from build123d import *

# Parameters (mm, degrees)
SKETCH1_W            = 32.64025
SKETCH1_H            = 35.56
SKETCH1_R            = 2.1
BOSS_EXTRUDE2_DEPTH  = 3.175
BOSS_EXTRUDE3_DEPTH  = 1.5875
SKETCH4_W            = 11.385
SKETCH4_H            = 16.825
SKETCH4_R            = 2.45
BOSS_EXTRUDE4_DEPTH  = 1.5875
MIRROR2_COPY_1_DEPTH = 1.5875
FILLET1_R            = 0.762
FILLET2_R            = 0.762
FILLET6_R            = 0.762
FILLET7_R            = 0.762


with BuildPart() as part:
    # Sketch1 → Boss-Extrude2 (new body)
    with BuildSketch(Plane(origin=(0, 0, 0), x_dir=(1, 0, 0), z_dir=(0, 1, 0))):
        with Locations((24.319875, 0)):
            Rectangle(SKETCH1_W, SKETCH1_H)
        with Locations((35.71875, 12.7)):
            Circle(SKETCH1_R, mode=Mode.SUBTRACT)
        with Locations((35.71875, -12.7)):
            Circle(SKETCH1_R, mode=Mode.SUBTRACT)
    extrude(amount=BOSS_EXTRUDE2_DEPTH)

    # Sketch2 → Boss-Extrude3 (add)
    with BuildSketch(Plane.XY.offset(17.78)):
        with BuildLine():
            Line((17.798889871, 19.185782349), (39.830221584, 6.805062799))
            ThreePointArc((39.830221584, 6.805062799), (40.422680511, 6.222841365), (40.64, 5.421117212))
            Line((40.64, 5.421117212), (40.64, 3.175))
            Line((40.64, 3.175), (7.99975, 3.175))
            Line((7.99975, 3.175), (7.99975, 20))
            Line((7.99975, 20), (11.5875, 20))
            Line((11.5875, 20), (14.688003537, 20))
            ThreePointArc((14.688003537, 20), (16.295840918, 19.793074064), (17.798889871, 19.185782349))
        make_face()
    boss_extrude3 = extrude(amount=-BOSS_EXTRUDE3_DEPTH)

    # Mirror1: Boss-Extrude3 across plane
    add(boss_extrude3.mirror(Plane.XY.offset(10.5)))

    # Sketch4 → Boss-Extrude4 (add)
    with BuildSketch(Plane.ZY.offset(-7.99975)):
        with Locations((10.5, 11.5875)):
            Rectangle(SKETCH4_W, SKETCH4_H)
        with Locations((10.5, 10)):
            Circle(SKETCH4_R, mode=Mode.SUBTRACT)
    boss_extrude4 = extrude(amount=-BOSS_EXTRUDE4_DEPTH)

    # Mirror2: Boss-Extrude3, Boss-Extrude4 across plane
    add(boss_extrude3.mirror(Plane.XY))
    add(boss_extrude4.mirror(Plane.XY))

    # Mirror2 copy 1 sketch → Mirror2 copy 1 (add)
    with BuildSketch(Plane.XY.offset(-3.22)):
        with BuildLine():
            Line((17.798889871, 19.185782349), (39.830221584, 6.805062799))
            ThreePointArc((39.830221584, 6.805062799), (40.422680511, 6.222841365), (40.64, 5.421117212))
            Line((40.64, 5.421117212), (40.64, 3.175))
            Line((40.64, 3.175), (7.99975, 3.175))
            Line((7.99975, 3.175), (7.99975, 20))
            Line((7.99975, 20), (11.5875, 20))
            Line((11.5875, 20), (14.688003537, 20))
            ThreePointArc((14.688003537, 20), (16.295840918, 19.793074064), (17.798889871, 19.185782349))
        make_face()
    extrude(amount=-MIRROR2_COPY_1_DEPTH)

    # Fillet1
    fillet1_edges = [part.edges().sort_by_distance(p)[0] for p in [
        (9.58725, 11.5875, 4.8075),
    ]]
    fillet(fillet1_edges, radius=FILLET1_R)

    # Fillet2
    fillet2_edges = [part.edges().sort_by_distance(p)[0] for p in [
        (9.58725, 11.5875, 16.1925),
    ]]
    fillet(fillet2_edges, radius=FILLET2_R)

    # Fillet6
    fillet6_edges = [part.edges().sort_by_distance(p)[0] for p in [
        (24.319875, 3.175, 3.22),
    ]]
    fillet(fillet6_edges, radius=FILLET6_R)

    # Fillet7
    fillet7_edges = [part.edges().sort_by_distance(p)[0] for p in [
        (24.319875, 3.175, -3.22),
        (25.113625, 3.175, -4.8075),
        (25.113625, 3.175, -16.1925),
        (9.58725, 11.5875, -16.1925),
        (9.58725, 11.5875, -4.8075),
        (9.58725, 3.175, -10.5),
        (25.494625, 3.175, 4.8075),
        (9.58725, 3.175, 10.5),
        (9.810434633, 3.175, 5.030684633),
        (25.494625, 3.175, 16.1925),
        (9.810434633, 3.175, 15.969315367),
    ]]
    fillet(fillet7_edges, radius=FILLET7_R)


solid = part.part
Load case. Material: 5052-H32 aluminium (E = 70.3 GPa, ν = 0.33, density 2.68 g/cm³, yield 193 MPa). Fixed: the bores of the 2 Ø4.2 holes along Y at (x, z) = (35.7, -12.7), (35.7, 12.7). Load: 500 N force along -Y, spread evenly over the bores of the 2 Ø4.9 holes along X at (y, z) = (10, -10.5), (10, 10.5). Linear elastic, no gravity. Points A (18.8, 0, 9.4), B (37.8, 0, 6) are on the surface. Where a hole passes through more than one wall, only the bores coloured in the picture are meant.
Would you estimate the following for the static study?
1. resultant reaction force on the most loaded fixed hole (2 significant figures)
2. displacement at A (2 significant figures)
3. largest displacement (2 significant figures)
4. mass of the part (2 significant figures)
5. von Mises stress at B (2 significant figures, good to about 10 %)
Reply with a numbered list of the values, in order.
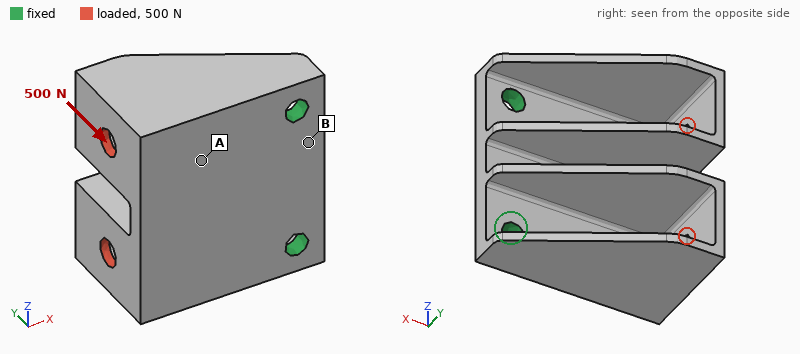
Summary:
1. 250 N
2. 0.082 mm
3. 0.18 mm
4. 18 g
5. 56 MPa
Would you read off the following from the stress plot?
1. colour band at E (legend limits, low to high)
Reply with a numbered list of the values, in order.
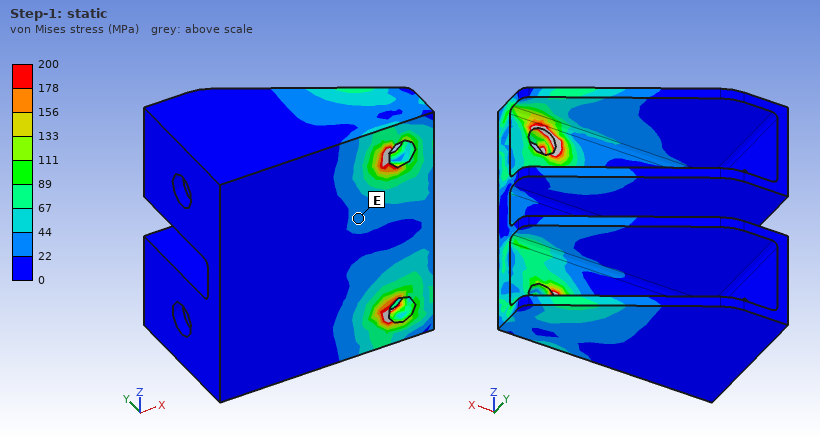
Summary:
1. 22 to 44 MPa
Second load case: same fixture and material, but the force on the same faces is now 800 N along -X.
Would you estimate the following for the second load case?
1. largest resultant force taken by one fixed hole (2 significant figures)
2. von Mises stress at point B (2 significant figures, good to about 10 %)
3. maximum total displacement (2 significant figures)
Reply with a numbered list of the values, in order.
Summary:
1. 400 N
2. 27 MPa
3. 96 µm
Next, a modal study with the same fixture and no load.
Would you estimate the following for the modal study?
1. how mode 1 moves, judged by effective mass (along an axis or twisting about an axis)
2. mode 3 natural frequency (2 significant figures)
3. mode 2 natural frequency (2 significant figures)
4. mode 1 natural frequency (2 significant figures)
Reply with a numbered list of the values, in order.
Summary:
1. along Y
2. 5800 Hz
3. 4300 Hz
4. 3400 Hz
